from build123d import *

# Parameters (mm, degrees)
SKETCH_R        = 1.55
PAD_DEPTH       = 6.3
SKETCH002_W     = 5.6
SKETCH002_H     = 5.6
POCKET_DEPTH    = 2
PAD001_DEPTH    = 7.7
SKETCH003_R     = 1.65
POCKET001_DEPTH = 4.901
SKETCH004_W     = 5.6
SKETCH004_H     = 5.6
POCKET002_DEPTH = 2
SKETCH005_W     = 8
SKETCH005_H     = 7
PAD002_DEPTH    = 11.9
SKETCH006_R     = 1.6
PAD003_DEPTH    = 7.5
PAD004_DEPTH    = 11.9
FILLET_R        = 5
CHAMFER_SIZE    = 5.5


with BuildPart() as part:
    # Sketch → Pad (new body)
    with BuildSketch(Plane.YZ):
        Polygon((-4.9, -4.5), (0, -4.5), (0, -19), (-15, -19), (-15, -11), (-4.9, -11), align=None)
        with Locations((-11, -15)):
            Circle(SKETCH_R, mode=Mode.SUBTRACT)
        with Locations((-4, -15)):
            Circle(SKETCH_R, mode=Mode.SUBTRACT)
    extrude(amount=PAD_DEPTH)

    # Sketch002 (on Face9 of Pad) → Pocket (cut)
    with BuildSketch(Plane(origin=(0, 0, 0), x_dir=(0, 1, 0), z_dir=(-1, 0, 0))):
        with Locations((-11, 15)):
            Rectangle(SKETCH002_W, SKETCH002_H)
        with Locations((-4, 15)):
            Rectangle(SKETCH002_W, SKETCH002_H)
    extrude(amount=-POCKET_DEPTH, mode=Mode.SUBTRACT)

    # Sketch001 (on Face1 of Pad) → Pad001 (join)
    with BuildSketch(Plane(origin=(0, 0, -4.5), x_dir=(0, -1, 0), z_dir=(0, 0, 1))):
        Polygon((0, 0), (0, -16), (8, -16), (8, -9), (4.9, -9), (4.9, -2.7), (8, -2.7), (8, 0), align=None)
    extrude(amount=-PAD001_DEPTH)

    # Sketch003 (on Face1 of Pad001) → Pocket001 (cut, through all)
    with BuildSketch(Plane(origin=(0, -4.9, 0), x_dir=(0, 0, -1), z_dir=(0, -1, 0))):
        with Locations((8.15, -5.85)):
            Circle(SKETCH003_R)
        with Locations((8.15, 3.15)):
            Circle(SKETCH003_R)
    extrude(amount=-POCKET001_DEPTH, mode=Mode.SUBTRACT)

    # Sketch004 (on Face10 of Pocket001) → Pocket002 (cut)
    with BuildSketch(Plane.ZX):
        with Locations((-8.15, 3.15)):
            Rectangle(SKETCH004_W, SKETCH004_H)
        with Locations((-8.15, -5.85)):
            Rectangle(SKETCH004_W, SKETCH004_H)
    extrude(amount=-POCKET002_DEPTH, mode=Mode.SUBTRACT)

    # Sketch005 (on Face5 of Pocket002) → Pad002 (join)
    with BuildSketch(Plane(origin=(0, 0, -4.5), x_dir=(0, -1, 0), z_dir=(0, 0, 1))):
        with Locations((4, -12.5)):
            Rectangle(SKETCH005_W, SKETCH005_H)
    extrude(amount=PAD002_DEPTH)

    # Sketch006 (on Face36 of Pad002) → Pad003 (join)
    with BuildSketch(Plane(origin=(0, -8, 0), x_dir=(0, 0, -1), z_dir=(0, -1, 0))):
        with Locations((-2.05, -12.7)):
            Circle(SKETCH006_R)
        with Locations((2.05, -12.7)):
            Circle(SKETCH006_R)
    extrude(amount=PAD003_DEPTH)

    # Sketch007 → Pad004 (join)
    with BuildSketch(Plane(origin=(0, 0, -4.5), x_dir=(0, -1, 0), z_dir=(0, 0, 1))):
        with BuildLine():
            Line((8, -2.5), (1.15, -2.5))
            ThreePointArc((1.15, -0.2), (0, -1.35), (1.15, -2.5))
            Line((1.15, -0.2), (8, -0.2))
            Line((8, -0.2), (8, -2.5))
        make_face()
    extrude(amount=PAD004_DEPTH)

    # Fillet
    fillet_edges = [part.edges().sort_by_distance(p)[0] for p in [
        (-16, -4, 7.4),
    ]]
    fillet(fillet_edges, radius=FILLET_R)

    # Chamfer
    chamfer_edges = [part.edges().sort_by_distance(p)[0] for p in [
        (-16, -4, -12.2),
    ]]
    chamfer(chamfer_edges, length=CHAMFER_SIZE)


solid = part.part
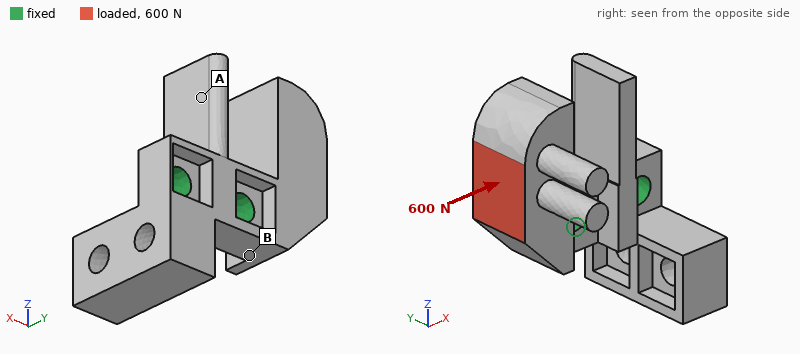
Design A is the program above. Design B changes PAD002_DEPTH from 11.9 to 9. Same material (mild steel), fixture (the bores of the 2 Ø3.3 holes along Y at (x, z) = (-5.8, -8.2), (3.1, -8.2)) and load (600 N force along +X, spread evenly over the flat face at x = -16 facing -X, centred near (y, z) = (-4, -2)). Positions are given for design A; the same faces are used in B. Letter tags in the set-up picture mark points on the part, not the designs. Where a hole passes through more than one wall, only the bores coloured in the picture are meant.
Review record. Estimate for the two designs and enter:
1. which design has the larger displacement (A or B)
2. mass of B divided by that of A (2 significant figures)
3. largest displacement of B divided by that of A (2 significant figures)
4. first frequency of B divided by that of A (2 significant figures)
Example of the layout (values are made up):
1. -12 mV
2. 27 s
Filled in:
1. A
2. 0.93
3. 0.74
4. 1.2
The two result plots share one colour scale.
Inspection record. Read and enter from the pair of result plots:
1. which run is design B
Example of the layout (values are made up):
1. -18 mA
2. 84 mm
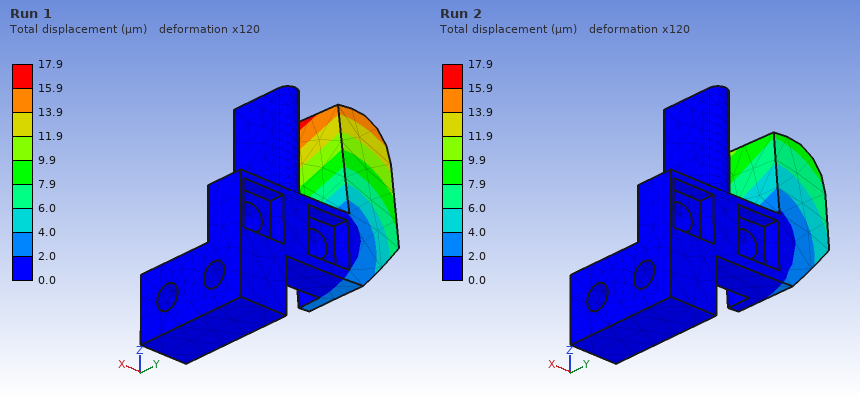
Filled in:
1. Run 2
